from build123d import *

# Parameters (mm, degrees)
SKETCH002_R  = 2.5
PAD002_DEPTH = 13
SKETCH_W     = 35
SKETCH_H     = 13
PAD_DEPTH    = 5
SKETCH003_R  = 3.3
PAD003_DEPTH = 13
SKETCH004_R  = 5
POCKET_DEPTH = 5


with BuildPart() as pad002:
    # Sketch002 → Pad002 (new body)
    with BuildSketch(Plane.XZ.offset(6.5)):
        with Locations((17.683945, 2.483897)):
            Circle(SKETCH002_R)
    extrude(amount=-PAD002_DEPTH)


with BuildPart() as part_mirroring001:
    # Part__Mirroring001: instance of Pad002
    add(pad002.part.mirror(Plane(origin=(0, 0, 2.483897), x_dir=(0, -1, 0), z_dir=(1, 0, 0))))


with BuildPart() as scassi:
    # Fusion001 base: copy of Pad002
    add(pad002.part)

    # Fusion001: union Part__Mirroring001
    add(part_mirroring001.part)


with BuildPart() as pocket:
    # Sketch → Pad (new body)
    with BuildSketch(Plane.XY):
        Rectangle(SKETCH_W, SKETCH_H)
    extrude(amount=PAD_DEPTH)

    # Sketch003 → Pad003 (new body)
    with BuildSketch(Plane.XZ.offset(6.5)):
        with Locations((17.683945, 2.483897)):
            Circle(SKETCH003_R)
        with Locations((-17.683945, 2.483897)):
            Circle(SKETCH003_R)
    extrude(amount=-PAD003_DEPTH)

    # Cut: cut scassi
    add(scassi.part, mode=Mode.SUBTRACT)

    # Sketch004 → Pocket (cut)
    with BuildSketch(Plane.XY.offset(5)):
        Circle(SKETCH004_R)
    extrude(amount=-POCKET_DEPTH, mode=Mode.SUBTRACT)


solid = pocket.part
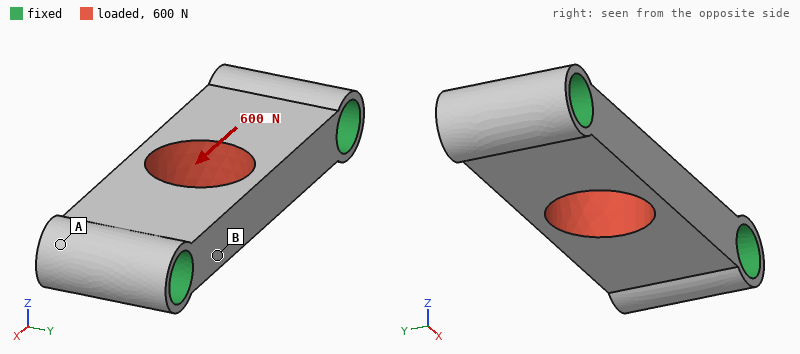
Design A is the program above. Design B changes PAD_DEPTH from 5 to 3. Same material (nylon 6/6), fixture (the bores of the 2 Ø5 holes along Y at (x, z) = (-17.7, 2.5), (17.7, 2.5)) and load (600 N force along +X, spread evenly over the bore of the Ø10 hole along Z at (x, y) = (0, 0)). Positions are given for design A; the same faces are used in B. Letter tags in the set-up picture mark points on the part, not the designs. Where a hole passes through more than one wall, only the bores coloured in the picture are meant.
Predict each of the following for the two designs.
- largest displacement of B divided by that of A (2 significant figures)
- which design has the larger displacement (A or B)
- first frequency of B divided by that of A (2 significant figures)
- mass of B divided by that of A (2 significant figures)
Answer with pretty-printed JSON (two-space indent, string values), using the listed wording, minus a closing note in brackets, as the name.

{
  "largest displacement of B divided by that of A": "1.7",
  "which design has the larger displacement": "B",
  "first frequency of B divided by that of A": "0.72",
  "mass of B divided by that of A": "0.68"
}
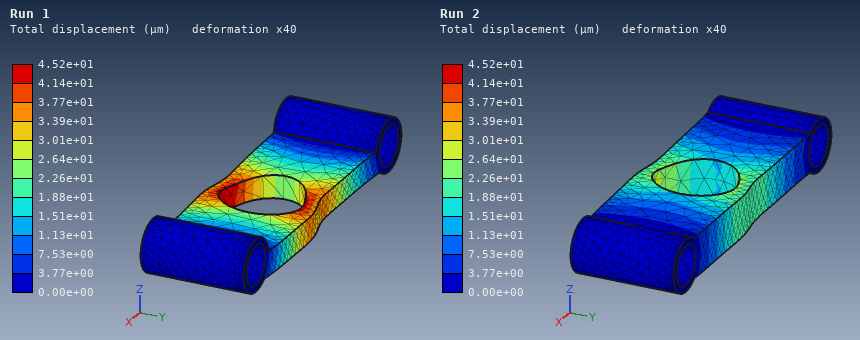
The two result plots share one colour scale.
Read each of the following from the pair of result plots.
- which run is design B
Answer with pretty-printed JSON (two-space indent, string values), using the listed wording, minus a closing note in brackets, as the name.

{
  "which run is design B": "Run 1"
}
